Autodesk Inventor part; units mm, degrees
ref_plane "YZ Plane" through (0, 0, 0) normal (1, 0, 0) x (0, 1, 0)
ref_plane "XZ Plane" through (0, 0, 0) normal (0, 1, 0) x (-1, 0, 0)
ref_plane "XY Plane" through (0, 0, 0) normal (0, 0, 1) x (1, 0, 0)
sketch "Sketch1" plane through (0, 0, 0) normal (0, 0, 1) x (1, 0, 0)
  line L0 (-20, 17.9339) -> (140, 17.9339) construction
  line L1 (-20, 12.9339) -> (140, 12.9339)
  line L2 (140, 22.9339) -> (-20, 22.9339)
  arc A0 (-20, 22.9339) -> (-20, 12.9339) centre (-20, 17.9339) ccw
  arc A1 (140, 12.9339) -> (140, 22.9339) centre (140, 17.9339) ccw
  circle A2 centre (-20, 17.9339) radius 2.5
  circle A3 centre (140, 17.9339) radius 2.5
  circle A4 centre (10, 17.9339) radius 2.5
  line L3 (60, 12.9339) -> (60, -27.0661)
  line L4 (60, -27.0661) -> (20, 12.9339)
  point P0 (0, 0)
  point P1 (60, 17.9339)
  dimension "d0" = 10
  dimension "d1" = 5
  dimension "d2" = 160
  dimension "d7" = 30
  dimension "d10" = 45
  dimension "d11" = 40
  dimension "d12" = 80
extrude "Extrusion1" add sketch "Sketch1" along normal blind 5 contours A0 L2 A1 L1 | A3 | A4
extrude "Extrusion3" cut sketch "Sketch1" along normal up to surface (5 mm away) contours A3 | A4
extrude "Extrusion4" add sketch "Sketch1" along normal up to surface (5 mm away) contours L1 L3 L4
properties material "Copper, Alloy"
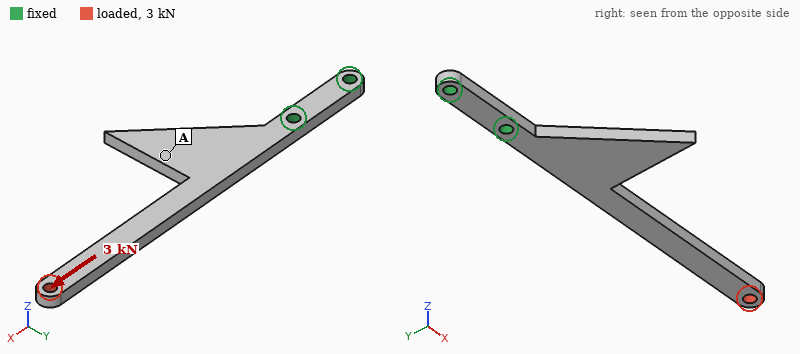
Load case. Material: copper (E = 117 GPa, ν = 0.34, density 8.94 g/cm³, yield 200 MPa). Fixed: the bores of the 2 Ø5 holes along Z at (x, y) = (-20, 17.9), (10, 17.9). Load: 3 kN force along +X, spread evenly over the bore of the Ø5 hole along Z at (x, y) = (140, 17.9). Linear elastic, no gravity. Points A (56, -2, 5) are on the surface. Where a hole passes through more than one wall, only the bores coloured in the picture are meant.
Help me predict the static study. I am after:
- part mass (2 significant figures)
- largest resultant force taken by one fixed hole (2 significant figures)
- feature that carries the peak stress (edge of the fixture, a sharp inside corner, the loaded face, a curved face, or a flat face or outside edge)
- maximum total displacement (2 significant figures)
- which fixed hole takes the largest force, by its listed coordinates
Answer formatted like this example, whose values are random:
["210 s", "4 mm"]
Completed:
["110 g", "3.0 kN", "the loaded face", "0.15 mm", "(10, 17.9)"]
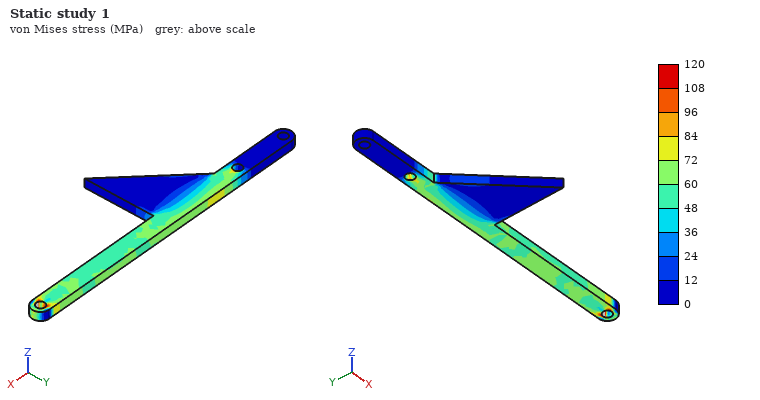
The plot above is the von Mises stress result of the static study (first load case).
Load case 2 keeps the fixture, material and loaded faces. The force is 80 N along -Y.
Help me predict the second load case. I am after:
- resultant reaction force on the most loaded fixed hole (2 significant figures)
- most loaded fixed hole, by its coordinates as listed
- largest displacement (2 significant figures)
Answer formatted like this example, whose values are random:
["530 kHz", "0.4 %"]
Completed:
["140 N", "(10, 17.9)", "0.83 mm"]
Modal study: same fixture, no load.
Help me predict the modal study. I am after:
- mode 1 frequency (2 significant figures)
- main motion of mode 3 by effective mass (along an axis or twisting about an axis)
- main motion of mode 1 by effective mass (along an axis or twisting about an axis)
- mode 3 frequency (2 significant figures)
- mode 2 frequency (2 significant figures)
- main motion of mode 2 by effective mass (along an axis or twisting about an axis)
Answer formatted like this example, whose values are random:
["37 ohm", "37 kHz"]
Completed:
["190 Hz", "along Z", "along Z", "750 Hz", "400 Hz", "along Y"]
